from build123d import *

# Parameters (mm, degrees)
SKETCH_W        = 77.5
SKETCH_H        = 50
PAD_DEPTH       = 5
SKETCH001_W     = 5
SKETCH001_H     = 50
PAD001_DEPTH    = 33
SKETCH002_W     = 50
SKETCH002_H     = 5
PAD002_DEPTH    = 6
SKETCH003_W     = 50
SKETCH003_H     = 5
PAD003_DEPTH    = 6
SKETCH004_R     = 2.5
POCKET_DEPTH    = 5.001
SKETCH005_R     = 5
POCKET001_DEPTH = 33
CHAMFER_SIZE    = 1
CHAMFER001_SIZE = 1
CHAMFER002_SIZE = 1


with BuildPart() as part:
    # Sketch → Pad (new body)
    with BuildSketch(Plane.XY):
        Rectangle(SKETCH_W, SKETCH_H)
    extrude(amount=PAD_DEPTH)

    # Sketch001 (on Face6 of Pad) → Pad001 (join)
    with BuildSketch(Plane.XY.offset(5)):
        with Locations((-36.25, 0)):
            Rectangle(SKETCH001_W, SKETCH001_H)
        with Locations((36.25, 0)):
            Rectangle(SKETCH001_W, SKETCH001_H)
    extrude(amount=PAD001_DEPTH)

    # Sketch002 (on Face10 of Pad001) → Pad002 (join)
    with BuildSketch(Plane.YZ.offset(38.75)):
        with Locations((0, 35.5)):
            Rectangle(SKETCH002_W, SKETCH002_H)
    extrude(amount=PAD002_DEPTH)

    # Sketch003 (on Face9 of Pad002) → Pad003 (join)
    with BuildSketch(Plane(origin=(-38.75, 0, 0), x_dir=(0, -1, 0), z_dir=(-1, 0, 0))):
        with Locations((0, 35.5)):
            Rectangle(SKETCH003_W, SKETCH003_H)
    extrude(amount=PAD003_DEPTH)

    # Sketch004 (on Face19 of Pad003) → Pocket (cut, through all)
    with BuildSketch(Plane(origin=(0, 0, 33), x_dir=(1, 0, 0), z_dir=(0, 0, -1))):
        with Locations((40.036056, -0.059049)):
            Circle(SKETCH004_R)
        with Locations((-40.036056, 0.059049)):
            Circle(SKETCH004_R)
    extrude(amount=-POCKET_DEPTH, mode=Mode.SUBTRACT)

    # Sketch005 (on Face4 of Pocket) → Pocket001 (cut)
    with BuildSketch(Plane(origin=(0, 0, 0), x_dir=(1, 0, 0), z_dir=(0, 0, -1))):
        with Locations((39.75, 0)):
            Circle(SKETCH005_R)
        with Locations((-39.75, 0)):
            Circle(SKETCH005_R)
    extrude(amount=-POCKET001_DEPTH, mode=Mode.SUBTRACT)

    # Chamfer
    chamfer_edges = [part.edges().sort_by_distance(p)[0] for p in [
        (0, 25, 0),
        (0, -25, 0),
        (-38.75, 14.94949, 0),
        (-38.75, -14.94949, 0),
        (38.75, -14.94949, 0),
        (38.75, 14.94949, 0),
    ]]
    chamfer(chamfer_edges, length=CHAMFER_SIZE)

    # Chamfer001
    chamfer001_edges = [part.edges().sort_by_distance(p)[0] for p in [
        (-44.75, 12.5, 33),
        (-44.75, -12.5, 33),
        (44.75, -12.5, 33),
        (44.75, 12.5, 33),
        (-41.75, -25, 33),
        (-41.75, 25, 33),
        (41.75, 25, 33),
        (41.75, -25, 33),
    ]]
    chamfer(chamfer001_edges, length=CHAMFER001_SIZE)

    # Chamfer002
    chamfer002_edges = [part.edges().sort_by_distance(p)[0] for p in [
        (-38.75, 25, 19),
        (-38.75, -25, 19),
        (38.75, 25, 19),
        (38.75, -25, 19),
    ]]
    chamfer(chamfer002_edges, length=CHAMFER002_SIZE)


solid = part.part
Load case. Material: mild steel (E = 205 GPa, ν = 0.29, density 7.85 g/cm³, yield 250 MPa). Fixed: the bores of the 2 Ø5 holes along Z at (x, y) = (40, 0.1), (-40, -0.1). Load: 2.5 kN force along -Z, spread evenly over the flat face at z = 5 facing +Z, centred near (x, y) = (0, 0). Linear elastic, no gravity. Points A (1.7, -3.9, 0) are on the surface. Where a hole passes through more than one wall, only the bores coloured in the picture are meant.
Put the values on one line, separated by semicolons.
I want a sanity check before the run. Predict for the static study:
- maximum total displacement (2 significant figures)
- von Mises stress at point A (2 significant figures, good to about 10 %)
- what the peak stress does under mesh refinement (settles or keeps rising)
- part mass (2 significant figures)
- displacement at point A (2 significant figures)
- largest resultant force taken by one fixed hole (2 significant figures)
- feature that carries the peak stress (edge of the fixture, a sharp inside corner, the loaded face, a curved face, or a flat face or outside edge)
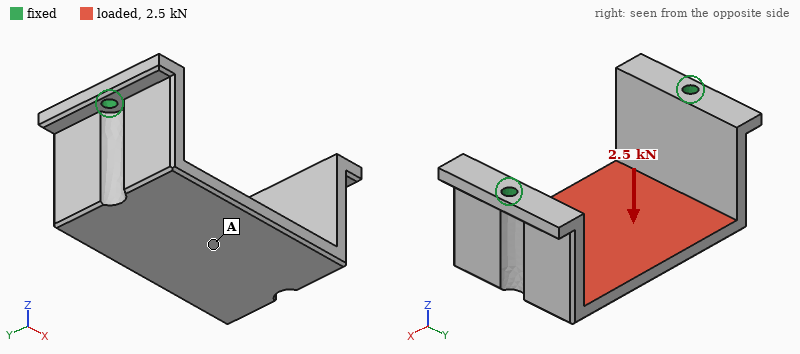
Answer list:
50 µm; 51 MPa; keeps rising; 290 g; 45 µm; 1.4 kN; edge of the fixture
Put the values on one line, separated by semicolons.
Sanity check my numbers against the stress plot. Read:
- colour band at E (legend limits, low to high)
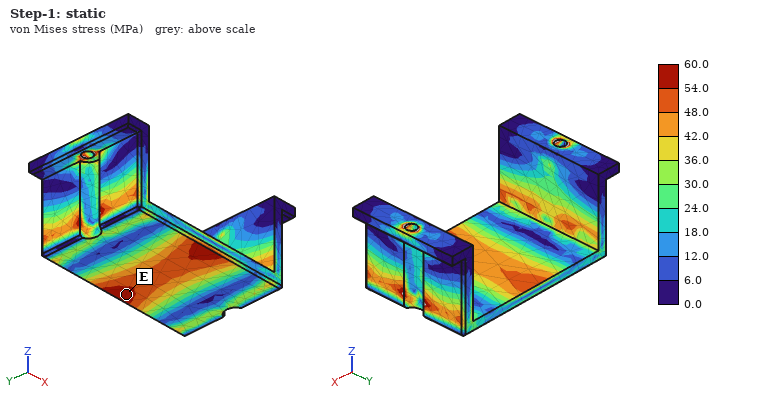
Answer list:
54.0 to 60.0 MPa
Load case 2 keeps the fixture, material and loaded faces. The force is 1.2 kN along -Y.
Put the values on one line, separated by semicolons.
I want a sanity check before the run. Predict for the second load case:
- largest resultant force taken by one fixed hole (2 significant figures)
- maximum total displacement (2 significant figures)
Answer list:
600 N; 56 µm
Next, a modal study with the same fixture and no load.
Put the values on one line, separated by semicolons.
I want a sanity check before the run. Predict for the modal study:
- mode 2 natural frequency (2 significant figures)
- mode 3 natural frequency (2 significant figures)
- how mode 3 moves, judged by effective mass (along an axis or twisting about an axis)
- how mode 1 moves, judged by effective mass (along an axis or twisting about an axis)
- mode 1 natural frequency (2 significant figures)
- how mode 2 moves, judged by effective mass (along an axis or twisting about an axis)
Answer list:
1800 Hz; 2500 Hz; twisting about Z; along Y; 1700 Hz; along X
